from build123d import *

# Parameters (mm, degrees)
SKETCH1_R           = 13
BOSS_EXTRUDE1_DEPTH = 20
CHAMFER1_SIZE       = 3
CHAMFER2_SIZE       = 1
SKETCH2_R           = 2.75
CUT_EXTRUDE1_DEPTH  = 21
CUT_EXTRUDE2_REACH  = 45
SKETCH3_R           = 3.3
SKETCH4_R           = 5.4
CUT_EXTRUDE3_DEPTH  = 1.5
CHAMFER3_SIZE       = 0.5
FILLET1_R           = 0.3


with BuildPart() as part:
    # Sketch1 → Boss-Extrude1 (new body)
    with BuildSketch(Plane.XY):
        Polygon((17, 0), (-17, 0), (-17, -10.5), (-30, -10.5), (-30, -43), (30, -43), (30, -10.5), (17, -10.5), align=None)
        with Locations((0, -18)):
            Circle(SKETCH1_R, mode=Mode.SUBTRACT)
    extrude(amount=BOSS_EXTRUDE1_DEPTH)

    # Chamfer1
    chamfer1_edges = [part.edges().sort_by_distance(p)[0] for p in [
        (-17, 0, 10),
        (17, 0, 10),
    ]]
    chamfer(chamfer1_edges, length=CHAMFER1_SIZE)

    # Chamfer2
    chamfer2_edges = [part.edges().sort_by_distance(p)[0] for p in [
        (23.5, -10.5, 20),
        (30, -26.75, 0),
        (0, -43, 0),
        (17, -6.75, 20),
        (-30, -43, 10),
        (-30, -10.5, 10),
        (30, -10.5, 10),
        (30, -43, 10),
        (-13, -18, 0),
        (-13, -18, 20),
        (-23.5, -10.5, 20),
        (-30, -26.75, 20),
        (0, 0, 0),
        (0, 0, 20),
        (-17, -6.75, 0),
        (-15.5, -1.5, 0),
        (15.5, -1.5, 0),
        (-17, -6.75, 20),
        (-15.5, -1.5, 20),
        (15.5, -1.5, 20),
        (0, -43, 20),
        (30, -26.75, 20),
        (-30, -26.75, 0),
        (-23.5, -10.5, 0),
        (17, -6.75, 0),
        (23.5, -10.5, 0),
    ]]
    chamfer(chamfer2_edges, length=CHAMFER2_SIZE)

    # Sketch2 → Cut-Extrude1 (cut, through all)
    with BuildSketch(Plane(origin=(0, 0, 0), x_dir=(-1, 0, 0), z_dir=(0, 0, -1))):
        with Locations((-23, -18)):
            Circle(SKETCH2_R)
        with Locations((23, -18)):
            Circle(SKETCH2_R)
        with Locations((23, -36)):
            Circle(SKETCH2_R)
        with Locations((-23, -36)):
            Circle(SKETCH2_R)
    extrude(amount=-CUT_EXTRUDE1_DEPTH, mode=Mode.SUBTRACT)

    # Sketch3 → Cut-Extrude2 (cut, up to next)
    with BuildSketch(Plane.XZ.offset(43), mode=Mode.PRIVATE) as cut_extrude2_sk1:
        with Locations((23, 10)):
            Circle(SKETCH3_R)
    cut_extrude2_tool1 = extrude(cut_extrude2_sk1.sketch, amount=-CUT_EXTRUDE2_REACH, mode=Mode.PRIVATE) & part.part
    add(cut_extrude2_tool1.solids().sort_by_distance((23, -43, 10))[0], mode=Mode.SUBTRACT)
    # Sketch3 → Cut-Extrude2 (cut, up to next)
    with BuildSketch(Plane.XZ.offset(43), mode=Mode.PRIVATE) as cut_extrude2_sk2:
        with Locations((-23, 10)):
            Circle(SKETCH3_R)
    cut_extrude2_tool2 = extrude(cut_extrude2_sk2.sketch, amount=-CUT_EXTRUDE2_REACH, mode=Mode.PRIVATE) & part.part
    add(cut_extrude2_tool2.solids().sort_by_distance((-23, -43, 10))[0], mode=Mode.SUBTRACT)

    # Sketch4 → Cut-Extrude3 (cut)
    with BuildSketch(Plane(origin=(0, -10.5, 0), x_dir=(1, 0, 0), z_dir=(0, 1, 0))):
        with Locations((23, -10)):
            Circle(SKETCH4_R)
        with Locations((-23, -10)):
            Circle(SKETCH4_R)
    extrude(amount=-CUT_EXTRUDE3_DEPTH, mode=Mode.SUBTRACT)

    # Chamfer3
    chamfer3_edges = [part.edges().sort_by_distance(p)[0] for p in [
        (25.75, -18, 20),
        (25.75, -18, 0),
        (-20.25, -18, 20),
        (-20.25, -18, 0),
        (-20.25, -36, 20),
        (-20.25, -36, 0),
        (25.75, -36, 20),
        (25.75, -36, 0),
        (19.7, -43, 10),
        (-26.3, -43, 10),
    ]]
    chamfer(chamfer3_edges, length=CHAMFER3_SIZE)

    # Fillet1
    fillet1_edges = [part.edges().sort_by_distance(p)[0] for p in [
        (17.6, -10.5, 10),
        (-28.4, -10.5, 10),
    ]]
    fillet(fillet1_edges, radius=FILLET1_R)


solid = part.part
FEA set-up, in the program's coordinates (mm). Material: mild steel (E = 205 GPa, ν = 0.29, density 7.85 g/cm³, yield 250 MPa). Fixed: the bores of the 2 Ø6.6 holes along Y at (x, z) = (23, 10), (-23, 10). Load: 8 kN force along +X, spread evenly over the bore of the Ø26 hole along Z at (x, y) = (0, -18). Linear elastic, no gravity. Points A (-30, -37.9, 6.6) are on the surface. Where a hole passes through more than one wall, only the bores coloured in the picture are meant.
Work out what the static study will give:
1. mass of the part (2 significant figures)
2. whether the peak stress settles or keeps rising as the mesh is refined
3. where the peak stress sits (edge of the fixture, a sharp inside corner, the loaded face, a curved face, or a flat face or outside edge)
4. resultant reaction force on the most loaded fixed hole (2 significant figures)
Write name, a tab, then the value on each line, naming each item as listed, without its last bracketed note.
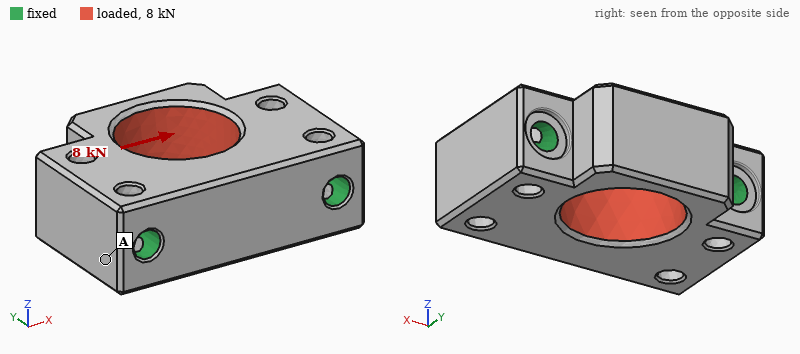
mass of the part	250 g
whether the peak stress settles or keeps rising as the mesh is refined	keeps rising
where the peak stress sits	a sharp inside corner
resultant reaction force on the most loaded fixed hole	4.0 kN
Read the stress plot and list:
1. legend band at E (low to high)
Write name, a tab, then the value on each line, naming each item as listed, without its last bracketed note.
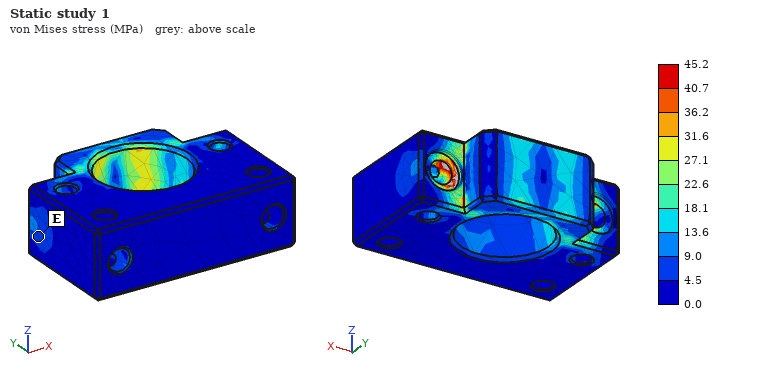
legend band at E	4.5 to 9.0 MPa
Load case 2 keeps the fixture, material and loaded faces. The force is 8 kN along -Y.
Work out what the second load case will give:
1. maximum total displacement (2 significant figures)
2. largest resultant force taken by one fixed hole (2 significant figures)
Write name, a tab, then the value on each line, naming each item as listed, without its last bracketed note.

maximum total displacement	3.3 µm
largest resultant force taken by one fixed hole	4.1 kN
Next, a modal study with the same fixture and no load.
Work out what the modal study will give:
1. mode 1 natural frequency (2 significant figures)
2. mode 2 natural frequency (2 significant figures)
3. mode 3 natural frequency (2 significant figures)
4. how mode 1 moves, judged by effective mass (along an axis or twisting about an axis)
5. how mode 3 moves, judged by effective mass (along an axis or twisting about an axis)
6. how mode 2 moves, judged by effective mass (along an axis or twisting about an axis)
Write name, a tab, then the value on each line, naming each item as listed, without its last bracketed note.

mode 1 natural frequency	16 kHz
mode 2 natural frequency	23 kHz
mode 3 natural frequency	26 kHz
how mode 1 moves, judged by effective mass	along Z
how mode 3 moves, judged by effective mass	along Z
how mode 2 moves, judged by effective mass	along X
